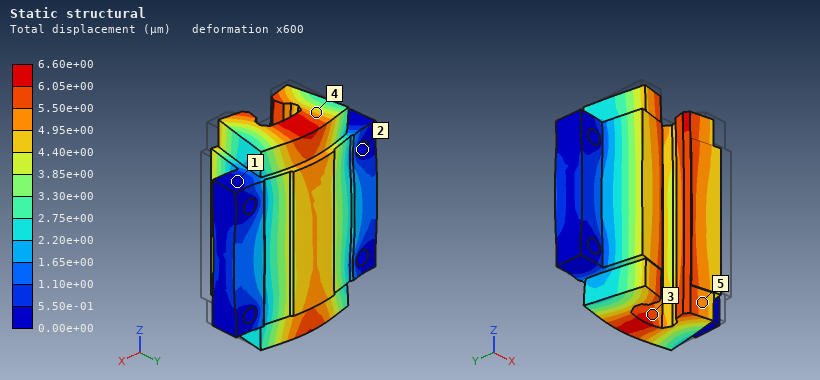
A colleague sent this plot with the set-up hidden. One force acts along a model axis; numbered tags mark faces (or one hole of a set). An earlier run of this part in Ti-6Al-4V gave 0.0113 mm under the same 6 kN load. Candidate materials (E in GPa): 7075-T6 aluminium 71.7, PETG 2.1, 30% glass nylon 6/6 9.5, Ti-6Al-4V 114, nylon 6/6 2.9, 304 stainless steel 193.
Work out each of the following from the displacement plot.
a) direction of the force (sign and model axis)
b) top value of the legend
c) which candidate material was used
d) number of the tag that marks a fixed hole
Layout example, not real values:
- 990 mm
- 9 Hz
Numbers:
- +Y
- 6.60e+00 µm
- 304 stainless steel
- 2
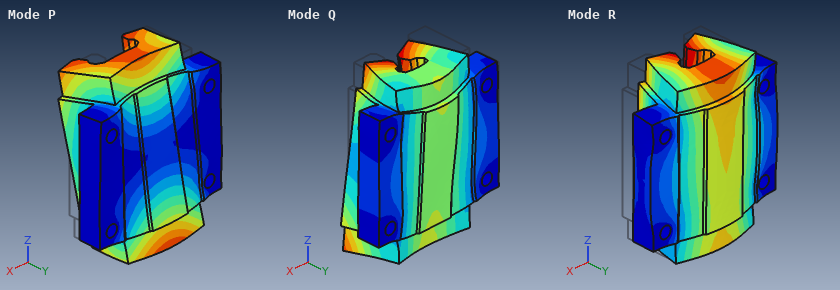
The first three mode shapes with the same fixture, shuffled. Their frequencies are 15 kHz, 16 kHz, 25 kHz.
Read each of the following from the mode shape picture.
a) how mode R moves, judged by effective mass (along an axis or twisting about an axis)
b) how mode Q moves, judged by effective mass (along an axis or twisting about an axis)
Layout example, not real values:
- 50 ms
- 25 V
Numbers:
- along Y
- along Z
